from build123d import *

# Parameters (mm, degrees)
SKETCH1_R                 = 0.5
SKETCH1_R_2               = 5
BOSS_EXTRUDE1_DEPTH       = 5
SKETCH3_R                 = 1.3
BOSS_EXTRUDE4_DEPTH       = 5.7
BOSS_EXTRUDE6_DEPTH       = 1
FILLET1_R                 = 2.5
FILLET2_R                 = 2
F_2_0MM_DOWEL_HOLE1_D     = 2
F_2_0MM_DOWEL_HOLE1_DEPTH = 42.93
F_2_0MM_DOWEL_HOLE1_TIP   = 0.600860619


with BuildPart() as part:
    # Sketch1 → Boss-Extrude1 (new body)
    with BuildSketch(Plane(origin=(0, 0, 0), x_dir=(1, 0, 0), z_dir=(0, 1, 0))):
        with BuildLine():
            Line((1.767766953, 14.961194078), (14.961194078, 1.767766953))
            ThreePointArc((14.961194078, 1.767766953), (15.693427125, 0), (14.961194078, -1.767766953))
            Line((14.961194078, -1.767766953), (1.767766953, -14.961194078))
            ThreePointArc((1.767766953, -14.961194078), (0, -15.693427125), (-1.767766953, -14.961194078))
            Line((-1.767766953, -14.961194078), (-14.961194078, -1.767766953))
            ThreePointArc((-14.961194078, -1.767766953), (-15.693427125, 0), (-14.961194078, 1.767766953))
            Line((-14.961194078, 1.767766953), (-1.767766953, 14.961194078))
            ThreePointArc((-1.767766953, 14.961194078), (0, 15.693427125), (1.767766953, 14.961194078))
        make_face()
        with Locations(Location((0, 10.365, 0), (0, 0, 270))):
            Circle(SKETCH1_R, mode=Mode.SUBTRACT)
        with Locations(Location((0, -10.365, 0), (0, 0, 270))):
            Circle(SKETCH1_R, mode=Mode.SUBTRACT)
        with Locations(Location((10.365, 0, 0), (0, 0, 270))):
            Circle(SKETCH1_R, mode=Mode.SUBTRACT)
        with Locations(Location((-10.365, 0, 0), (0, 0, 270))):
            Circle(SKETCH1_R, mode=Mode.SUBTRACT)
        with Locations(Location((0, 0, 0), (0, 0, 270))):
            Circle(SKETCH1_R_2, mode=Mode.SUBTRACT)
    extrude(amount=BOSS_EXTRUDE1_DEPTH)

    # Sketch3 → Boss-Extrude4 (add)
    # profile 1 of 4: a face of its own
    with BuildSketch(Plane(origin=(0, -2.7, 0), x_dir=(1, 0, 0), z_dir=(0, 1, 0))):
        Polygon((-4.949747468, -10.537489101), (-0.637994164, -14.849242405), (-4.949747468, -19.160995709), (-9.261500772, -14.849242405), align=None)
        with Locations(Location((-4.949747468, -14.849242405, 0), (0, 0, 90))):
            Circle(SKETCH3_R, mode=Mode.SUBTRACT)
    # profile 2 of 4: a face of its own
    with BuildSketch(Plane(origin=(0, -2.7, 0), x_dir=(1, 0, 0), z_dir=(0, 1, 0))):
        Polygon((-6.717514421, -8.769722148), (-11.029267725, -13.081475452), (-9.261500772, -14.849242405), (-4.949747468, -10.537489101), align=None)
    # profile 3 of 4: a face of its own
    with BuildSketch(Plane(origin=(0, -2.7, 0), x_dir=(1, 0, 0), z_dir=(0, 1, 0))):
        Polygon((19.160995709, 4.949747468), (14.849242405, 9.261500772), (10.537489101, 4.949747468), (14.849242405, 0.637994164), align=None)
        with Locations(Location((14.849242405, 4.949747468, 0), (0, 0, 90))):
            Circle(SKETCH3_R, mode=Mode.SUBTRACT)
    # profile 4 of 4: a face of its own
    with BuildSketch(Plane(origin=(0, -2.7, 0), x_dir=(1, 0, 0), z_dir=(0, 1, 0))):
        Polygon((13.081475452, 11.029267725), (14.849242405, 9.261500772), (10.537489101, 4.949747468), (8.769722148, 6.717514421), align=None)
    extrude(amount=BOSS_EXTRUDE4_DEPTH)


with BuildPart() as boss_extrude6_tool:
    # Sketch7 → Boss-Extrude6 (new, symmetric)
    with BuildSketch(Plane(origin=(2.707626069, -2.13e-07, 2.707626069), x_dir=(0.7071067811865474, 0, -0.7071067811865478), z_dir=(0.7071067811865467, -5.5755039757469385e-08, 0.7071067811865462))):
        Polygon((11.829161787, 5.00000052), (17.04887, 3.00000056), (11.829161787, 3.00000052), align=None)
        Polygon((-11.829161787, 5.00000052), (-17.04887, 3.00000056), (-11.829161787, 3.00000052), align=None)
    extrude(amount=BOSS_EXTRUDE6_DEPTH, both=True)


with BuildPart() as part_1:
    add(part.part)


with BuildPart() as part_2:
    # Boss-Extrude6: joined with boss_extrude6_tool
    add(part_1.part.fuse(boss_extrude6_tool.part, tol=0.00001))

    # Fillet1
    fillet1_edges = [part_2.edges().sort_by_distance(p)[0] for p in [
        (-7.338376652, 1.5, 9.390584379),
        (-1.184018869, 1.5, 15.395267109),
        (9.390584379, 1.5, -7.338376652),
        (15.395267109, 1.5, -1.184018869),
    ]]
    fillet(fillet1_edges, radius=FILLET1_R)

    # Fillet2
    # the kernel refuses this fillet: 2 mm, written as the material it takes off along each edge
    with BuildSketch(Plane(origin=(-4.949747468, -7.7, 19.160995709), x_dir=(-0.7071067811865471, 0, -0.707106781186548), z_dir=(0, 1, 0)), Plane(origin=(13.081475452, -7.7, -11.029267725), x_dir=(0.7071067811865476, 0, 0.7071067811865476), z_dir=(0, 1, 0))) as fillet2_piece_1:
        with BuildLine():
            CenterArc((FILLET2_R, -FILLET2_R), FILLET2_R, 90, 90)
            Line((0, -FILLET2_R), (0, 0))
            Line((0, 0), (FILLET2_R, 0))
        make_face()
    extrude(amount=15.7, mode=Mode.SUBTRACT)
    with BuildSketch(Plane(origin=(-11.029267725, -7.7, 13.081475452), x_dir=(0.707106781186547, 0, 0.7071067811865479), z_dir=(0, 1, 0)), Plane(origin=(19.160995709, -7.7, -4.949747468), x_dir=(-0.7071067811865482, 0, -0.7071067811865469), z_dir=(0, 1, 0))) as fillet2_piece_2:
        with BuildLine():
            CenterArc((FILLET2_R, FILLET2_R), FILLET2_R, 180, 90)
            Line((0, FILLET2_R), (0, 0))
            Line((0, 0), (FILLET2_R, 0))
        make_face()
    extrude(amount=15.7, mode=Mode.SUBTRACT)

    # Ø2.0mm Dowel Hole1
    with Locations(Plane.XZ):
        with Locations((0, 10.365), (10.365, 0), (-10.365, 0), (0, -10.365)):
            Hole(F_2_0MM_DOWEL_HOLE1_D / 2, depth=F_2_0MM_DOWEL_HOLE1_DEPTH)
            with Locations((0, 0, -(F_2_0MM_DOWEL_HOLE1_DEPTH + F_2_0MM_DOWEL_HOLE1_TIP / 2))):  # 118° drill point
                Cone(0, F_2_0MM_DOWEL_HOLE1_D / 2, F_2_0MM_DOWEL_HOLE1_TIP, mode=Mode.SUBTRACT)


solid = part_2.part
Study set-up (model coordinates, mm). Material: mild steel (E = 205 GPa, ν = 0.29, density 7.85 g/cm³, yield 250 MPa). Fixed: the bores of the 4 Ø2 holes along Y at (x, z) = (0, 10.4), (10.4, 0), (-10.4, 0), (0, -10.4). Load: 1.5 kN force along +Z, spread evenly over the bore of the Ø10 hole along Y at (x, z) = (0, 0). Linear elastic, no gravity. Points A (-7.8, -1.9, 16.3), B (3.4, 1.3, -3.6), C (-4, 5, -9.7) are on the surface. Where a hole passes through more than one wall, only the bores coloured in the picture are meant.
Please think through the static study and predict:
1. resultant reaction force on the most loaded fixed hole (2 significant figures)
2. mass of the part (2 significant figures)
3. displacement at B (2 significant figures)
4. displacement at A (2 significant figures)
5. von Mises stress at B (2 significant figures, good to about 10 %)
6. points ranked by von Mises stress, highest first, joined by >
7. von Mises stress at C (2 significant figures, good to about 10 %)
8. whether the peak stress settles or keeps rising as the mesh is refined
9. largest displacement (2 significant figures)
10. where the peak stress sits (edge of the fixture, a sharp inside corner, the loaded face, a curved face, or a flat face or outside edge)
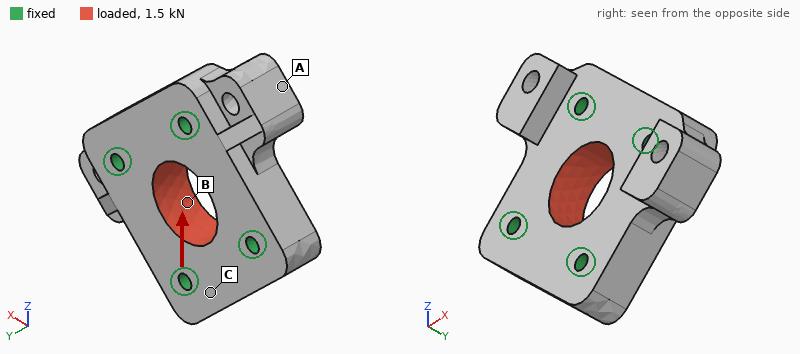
460 N
22 g
0.50 µm
0.32 µm
13 MPa
B > C > A
6.5 MPa
keeps rising
0.56 µm
edge of the fixture
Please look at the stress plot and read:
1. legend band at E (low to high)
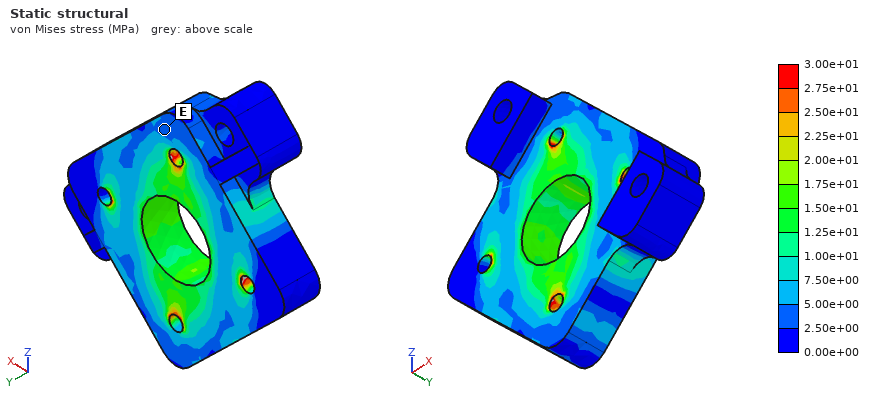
2.50e+00 to 5.00e+00 MPa
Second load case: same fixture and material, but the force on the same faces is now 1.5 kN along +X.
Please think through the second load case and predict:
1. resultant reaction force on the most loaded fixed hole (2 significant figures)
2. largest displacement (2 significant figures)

460 N
0.56 µm
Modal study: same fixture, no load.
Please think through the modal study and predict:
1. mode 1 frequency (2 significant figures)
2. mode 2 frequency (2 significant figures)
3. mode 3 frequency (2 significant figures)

31 kHz
32 kHz
51 kHz
